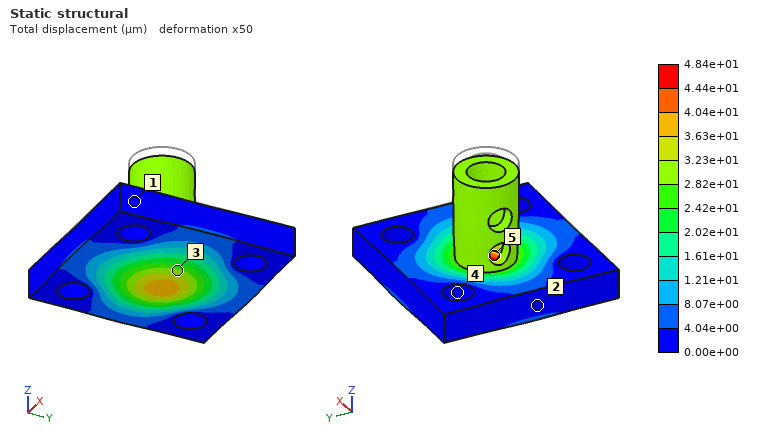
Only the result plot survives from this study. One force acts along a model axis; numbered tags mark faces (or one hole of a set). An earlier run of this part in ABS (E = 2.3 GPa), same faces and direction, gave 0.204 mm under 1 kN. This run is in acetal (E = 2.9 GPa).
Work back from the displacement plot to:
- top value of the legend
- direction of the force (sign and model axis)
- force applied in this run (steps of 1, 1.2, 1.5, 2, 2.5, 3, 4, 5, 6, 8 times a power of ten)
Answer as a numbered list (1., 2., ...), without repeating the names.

1. 4.84e+01 µm
2. -Z
3. 300 N
